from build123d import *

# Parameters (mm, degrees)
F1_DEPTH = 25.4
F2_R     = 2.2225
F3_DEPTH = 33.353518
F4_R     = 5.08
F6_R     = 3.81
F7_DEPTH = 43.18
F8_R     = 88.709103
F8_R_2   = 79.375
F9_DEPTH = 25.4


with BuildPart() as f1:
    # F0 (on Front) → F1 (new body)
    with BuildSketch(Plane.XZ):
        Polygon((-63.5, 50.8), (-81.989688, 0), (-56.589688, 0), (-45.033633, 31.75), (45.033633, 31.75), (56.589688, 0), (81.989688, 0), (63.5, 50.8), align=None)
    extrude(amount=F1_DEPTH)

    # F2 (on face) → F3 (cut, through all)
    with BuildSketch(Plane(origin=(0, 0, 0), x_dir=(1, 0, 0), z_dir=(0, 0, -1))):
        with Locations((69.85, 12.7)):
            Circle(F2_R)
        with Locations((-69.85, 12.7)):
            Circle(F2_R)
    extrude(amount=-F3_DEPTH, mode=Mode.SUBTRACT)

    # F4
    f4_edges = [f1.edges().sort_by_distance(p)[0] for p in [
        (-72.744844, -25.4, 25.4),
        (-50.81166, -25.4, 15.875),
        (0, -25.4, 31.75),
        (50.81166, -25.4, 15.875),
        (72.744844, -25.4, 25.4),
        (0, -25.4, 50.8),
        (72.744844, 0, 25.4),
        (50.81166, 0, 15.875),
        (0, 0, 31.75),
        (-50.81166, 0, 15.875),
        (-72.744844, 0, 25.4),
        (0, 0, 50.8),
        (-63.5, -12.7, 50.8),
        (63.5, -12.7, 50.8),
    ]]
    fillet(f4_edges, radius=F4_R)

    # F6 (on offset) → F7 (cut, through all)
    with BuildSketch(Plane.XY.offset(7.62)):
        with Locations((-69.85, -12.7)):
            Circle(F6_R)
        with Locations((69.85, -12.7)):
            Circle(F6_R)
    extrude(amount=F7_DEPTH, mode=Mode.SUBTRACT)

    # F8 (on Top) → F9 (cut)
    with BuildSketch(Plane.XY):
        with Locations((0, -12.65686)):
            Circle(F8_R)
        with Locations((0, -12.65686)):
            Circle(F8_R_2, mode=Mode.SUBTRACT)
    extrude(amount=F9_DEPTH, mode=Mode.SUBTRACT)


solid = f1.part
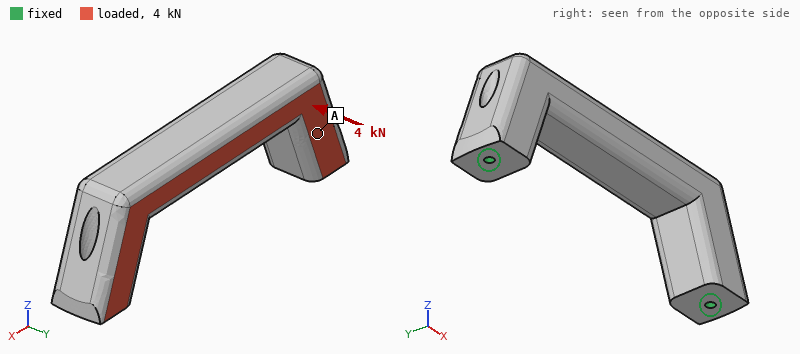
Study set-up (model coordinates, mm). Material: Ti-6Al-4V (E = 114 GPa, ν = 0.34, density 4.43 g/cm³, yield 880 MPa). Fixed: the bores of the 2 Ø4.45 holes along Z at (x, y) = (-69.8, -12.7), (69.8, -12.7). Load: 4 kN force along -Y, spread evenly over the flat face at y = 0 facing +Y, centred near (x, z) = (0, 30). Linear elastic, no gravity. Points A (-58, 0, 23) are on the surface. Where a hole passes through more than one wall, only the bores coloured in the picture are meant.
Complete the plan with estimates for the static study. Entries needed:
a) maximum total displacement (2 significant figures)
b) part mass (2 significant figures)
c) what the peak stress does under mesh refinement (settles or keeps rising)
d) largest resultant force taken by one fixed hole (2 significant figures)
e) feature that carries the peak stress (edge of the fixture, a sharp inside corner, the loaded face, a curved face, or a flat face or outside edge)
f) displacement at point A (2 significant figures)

0.13 mm
440 g
keeps rising
2.0 kN
edge of the fixture
0.055 mm
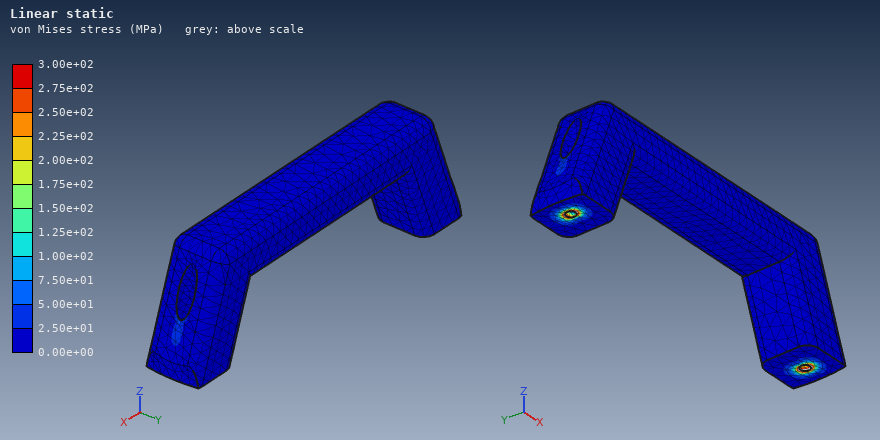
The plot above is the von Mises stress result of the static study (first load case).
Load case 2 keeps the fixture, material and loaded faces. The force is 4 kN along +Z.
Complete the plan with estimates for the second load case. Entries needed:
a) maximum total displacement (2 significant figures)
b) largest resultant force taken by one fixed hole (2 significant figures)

56 µm
2.2 kN
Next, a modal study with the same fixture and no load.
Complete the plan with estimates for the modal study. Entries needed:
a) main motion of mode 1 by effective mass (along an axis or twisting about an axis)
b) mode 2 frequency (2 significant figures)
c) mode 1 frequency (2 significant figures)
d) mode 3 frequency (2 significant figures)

along Y
3600 Hz
1500 Hz
3700 Hz
